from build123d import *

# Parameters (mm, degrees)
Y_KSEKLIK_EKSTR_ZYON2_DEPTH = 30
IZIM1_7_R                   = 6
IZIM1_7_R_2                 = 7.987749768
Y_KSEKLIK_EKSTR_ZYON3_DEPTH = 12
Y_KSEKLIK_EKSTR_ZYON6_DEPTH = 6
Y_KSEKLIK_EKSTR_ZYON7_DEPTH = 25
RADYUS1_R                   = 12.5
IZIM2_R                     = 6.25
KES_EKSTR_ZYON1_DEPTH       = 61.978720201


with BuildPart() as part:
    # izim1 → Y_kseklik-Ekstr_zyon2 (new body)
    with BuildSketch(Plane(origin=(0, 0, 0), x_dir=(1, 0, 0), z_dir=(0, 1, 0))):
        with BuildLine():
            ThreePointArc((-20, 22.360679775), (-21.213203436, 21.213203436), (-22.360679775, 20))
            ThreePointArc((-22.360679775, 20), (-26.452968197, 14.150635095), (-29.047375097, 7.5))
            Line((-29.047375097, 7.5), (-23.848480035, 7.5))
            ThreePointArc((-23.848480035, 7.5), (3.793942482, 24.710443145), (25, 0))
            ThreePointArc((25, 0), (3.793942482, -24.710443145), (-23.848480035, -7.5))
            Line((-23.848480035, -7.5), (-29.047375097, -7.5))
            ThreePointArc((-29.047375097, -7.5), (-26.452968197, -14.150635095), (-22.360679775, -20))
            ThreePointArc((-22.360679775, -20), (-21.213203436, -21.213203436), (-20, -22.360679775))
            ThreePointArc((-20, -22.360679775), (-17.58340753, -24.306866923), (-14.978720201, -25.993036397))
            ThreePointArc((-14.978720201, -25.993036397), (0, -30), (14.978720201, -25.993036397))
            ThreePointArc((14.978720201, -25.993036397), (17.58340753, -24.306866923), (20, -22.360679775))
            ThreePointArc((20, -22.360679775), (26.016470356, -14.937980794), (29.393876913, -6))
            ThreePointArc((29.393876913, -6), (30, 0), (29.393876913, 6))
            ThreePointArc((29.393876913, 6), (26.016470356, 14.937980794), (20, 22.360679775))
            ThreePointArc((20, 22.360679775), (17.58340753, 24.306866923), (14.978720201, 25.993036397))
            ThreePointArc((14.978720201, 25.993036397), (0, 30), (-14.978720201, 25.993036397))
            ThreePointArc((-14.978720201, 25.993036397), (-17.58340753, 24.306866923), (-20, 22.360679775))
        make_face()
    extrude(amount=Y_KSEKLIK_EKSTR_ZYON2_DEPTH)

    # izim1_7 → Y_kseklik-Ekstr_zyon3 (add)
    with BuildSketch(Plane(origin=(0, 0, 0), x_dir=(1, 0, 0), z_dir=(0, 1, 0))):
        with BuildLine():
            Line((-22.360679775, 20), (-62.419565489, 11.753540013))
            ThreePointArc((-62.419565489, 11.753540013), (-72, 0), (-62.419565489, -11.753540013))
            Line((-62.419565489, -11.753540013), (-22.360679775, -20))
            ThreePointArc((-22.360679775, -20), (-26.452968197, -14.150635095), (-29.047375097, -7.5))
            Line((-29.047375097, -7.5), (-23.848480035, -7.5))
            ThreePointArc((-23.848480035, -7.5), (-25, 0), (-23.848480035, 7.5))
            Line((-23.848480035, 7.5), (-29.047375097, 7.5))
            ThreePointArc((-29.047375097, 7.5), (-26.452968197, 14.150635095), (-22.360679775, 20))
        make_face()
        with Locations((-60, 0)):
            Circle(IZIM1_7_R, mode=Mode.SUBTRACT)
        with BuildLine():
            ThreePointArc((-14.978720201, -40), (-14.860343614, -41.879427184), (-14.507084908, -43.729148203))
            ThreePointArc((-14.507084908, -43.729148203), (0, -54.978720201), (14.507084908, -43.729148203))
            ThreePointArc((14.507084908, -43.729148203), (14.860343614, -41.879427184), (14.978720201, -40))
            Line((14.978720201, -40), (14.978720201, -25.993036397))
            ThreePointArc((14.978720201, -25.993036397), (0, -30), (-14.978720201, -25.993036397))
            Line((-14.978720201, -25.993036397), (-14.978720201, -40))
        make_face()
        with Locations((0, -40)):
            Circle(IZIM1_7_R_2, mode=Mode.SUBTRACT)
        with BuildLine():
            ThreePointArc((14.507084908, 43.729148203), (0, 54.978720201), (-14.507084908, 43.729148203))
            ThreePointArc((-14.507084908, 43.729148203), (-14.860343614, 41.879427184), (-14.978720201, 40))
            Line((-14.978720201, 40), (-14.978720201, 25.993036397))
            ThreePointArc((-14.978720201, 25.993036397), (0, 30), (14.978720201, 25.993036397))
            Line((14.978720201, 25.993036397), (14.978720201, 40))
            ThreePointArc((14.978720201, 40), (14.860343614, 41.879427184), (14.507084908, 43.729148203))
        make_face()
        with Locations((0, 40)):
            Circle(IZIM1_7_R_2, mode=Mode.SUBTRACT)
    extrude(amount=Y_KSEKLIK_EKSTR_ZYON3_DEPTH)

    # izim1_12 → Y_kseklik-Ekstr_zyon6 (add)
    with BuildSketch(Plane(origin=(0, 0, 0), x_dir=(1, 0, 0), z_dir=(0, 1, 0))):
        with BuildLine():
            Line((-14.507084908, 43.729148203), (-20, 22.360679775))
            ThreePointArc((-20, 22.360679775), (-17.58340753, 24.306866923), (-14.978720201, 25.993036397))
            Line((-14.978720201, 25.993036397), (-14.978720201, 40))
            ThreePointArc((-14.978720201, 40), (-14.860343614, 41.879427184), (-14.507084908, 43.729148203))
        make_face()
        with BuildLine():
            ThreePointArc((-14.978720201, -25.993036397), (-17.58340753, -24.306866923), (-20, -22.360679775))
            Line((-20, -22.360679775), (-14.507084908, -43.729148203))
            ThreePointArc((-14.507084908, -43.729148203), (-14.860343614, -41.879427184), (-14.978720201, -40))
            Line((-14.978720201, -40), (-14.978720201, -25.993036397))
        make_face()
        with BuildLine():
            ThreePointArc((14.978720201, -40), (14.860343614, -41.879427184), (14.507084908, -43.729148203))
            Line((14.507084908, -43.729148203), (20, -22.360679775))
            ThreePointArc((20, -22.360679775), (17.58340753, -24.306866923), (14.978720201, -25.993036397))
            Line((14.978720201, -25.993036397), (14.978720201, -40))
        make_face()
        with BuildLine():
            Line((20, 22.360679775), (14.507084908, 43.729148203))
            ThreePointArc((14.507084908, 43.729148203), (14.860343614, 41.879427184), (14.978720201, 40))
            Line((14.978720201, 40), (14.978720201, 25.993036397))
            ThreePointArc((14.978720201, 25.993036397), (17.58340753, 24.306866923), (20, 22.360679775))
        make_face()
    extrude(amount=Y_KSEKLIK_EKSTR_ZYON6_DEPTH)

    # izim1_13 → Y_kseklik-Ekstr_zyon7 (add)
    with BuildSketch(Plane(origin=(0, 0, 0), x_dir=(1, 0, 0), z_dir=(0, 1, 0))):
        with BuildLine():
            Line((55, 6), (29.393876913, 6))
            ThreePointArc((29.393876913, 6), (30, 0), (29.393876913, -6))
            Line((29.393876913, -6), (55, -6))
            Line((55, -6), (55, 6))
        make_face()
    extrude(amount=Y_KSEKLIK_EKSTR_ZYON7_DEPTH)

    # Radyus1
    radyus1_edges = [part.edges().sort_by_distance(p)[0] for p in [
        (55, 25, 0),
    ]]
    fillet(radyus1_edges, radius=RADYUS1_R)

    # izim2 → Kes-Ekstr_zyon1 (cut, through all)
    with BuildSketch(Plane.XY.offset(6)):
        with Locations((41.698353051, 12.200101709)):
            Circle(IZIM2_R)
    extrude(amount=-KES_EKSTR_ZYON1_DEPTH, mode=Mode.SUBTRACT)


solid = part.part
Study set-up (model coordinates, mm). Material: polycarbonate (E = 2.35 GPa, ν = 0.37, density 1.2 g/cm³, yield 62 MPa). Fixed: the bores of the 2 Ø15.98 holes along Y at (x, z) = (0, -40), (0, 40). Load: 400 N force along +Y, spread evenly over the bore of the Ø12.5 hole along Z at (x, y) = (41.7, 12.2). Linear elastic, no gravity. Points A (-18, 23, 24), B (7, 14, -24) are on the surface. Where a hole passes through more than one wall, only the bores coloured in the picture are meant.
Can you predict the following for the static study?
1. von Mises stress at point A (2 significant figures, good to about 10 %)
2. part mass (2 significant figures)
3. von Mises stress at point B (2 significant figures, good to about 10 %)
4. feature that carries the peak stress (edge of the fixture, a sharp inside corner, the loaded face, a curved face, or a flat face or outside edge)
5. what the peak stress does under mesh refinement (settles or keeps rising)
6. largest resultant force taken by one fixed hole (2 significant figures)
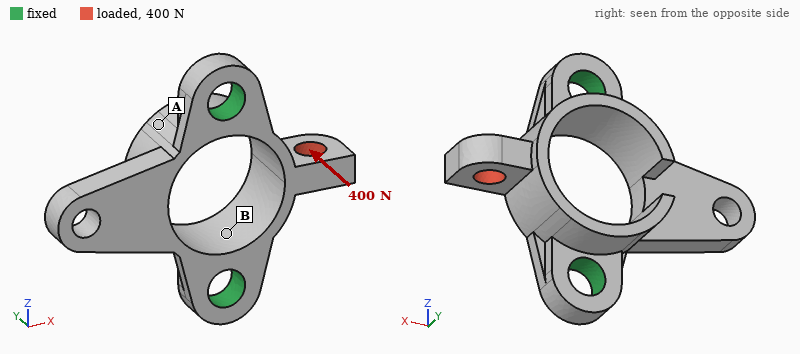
3.1 MPa
68 g
8.8 MPa
edge of the fixture
keeps rising
230 N
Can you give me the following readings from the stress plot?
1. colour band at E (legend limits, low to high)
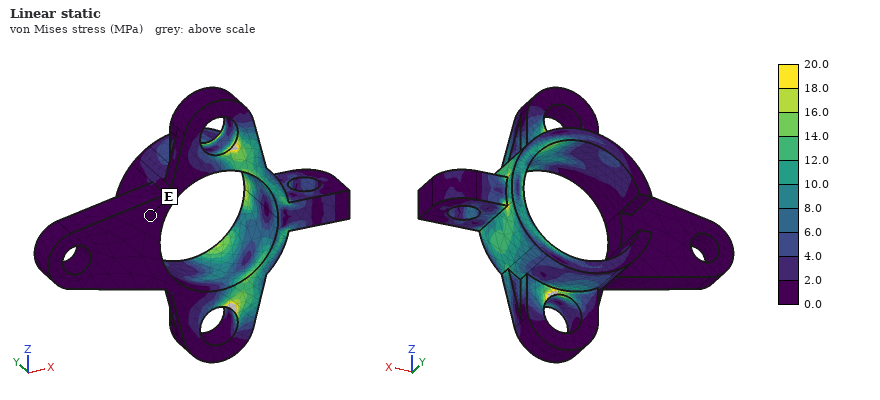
0.0 to 2.0 MPa
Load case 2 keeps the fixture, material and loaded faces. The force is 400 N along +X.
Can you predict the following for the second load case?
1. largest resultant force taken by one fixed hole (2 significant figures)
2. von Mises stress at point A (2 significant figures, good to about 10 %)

290 N
0.63 MPa
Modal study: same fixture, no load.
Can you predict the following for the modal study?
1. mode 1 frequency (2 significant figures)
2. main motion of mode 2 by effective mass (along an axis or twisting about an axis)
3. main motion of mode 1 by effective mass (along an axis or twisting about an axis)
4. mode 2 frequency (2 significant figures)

620 Hz
along Y
along Y
990 Hz
